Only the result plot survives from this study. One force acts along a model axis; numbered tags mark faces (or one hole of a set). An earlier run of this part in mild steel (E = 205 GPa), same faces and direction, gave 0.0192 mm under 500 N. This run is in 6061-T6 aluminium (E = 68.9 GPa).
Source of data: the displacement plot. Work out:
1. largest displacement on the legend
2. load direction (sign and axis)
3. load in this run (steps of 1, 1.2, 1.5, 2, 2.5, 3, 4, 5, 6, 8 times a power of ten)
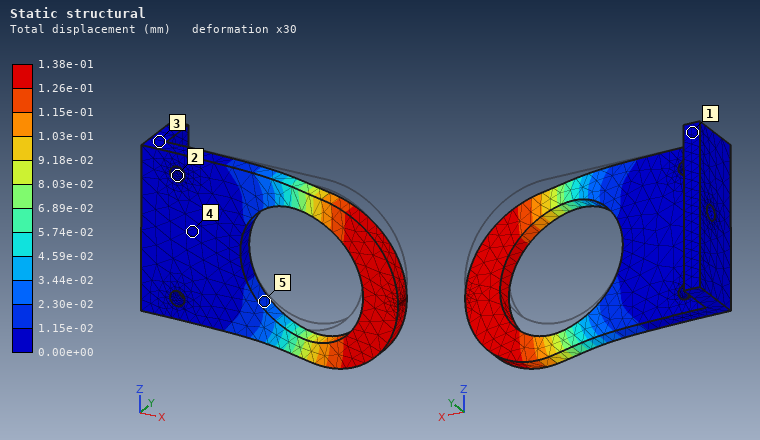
1.38e-01 mm
-Z
1.2 kN
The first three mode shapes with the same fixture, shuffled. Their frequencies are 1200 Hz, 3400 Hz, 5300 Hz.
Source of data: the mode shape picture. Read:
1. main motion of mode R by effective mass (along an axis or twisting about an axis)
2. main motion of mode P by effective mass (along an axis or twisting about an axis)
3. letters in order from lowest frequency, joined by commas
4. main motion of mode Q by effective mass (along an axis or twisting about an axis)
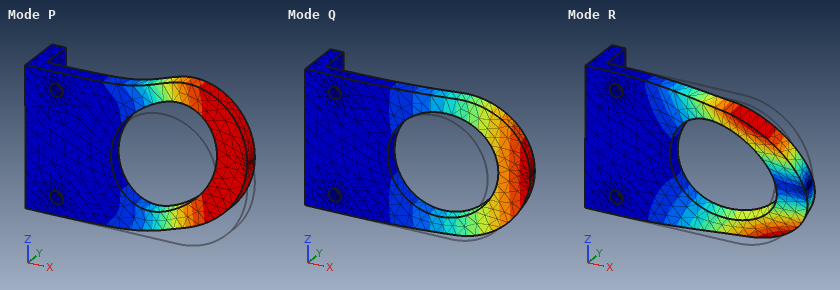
twisting about X
along Z
Q, R, P
along Y
